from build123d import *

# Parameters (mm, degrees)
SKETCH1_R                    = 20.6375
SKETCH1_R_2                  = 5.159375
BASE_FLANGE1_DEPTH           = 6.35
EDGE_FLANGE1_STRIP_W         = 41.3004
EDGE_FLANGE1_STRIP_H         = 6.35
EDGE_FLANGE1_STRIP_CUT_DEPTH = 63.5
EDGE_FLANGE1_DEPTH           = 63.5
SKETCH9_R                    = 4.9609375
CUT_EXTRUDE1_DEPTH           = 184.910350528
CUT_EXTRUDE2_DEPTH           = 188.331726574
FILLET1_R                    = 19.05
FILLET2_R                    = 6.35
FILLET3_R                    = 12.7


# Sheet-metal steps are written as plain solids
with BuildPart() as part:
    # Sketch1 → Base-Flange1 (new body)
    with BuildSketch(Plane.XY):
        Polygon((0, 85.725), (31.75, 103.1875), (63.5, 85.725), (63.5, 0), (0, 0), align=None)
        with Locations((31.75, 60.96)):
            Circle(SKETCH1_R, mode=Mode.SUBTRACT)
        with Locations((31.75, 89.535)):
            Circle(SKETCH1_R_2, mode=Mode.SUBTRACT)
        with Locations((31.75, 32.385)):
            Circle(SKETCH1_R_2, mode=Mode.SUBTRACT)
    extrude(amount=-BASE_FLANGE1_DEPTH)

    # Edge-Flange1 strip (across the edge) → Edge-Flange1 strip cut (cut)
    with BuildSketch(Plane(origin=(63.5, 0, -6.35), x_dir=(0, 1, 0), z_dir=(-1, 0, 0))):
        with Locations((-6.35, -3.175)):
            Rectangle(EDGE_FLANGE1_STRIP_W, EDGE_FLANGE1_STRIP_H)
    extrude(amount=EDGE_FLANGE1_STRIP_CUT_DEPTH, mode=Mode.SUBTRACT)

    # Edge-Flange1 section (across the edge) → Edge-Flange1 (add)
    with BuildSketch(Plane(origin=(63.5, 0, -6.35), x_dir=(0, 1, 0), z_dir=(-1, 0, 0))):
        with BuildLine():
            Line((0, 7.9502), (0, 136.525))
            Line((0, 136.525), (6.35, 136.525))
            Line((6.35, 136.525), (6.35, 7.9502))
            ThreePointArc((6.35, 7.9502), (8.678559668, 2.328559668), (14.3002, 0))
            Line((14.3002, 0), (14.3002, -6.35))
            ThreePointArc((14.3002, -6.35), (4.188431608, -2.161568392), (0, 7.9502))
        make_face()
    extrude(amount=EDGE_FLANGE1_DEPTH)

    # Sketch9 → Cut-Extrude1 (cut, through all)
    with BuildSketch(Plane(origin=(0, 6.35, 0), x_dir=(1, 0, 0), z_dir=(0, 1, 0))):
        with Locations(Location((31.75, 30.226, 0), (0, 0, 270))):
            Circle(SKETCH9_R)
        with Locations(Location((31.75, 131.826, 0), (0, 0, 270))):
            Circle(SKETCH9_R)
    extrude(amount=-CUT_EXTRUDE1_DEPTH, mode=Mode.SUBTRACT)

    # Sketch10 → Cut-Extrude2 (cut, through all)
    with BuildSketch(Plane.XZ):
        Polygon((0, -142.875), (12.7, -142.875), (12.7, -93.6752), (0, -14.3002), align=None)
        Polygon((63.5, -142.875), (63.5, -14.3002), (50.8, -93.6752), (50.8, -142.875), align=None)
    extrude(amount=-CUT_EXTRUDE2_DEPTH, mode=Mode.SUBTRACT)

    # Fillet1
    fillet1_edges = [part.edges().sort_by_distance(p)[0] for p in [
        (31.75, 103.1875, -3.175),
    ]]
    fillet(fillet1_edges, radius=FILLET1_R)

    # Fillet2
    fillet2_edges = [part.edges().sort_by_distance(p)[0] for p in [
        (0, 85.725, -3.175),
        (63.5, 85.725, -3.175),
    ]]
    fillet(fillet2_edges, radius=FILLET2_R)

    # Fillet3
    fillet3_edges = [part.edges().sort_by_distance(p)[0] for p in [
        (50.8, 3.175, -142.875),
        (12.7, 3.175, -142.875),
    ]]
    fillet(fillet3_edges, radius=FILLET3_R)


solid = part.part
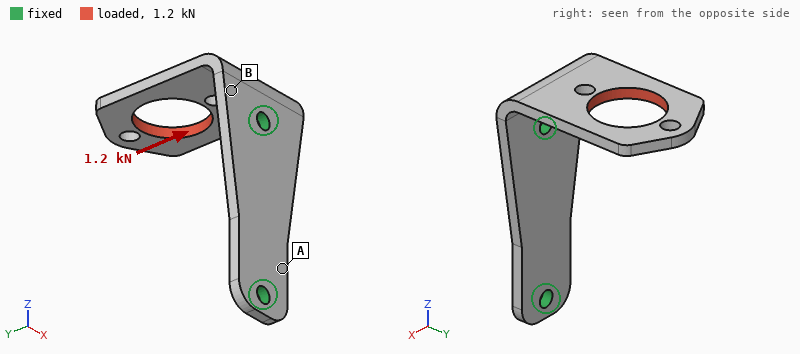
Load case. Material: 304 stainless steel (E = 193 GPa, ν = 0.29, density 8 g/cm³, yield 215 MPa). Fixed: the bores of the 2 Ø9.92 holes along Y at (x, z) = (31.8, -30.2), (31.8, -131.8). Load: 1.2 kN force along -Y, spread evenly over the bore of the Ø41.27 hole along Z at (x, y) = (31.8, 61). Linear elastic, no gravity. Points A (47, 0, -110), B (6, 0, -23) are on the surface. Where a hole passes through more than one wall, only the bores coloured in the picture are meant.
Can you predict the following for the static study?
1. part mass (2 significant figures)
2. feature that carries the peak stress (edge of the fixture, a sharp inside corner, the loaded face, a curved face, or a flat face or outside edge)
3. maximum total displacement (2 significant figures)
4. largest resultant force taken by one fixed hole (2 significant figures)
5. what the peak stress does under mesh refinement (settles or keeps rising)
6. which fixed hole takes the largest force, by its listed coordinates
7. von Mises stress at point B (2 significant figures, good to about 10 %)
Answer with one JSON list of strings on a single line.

["530 g", "edge of the fixture", "0.18 mm", "1.2 kN", "keeps rising", "(31.8, -30.2)", "31 MPa"]
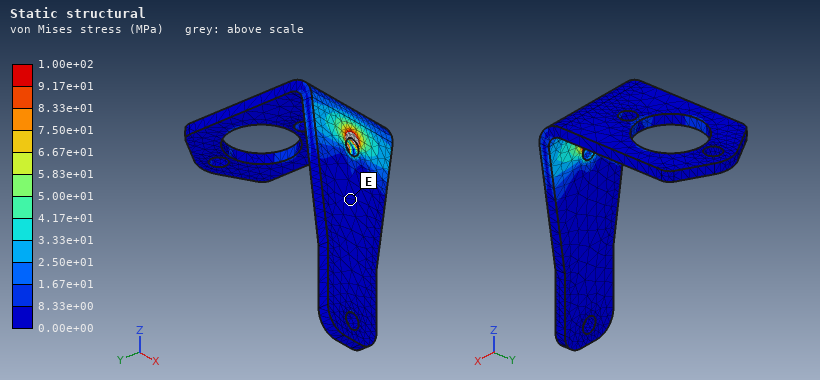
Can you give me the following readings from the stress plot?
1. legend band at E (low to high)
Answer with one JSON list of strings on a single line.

["0.00e+00 to 8.33e+00 MPa"]
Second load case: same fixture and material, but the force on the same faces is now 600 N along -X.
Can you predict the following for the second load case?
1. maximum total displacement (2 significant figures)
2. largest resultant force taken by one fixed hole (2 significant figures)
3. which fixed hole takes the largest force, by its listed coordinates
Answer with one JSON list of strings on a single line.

["0.20 mm", "710 N", "(31.8, -30.2)"]
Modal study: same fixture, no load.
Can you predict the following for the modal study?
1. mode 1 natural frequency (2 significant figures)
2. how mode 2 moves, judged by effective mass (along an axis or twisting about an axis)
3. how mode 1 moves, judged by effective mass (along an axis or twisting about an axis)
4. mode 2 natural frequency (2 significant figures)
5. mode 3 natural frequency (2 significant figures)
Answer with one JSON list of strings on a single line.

["490 Hz", "along X", "along Z", "820 Hz", "1700 Hz"]
